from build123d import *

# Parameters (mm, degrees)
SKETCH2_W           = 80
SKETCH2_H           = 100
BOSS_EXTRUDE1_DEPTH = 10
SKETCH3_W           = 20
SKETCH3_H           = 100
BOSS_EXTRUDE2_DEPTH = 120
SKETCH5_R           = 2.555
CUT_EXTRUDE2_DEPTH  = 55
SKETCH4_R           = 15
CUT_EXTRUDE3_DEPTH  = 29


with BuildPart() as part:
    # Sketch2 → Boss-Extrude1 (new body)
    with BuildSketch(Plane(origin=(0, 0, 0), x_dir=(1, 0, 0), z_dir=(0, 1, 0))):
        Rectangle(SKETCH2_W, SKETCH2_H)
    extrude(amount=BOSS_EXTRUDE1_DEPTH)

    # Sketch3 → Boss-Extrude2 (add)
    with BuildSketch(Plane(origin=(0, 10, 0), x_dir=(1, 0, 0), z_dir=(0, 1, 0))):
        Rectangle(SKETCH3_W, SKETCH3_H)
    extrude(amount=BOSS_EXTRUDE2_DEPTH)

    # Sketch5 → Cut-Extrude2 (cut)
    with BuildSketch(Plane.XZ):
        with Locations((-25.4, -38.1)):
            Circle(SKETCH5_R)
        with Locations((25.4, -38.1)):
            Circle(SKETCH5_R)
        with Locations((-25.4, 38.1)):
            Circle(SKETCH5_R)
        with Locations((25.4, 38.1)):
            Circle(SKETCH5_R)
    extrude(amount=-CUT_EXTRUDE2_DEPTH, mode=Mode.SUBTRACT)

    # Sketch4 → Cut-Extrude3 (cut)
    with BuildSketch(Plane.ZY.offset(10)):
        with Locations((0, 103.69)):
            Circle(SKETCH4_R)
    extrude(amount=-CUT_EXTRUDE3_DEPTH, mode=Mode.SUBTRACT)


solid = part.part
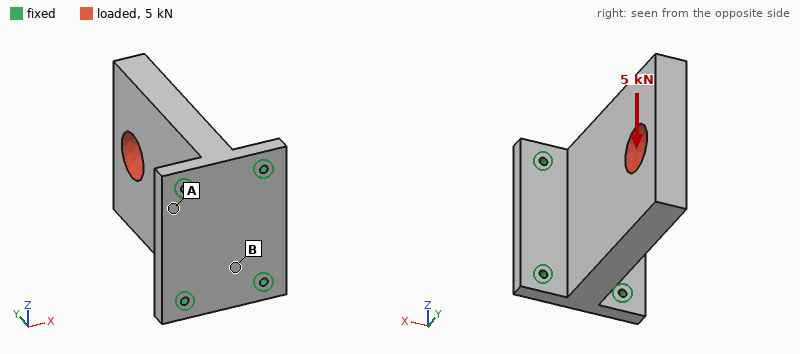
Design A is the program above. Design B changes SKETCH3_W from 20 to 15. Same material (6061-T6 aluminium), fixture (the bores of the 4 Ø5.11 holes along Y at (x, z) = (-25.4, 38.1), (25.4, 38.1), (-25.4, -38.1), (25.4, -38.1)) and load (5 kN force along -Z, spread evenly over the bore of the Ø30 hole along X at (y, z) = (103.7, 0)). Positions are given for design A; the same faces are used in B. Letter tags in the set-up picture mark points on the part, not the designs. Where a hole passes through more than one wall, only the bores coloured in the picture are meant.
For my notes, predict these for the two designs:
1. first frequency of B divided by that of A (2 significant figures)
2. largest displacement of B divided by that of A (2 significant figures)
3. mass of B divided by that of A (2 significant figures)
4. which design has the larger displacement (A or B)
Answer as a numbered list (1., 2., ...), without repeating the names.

1. 0.84
2. 1.2
3. 0.81
4. B
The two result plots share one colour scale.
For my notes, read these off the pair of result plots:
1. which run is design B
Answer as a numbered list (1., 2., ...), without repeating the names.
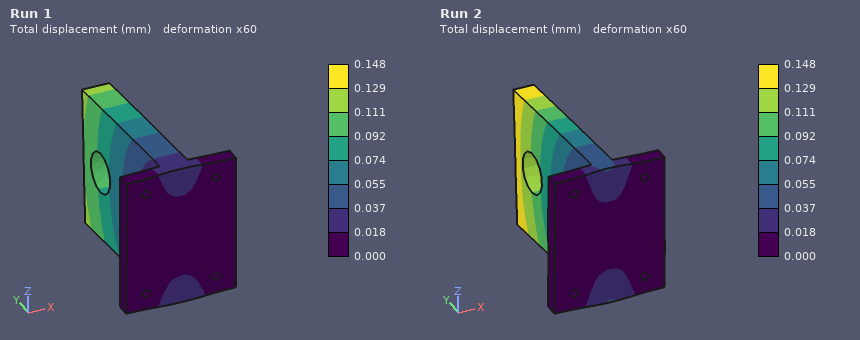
1. Run 2
